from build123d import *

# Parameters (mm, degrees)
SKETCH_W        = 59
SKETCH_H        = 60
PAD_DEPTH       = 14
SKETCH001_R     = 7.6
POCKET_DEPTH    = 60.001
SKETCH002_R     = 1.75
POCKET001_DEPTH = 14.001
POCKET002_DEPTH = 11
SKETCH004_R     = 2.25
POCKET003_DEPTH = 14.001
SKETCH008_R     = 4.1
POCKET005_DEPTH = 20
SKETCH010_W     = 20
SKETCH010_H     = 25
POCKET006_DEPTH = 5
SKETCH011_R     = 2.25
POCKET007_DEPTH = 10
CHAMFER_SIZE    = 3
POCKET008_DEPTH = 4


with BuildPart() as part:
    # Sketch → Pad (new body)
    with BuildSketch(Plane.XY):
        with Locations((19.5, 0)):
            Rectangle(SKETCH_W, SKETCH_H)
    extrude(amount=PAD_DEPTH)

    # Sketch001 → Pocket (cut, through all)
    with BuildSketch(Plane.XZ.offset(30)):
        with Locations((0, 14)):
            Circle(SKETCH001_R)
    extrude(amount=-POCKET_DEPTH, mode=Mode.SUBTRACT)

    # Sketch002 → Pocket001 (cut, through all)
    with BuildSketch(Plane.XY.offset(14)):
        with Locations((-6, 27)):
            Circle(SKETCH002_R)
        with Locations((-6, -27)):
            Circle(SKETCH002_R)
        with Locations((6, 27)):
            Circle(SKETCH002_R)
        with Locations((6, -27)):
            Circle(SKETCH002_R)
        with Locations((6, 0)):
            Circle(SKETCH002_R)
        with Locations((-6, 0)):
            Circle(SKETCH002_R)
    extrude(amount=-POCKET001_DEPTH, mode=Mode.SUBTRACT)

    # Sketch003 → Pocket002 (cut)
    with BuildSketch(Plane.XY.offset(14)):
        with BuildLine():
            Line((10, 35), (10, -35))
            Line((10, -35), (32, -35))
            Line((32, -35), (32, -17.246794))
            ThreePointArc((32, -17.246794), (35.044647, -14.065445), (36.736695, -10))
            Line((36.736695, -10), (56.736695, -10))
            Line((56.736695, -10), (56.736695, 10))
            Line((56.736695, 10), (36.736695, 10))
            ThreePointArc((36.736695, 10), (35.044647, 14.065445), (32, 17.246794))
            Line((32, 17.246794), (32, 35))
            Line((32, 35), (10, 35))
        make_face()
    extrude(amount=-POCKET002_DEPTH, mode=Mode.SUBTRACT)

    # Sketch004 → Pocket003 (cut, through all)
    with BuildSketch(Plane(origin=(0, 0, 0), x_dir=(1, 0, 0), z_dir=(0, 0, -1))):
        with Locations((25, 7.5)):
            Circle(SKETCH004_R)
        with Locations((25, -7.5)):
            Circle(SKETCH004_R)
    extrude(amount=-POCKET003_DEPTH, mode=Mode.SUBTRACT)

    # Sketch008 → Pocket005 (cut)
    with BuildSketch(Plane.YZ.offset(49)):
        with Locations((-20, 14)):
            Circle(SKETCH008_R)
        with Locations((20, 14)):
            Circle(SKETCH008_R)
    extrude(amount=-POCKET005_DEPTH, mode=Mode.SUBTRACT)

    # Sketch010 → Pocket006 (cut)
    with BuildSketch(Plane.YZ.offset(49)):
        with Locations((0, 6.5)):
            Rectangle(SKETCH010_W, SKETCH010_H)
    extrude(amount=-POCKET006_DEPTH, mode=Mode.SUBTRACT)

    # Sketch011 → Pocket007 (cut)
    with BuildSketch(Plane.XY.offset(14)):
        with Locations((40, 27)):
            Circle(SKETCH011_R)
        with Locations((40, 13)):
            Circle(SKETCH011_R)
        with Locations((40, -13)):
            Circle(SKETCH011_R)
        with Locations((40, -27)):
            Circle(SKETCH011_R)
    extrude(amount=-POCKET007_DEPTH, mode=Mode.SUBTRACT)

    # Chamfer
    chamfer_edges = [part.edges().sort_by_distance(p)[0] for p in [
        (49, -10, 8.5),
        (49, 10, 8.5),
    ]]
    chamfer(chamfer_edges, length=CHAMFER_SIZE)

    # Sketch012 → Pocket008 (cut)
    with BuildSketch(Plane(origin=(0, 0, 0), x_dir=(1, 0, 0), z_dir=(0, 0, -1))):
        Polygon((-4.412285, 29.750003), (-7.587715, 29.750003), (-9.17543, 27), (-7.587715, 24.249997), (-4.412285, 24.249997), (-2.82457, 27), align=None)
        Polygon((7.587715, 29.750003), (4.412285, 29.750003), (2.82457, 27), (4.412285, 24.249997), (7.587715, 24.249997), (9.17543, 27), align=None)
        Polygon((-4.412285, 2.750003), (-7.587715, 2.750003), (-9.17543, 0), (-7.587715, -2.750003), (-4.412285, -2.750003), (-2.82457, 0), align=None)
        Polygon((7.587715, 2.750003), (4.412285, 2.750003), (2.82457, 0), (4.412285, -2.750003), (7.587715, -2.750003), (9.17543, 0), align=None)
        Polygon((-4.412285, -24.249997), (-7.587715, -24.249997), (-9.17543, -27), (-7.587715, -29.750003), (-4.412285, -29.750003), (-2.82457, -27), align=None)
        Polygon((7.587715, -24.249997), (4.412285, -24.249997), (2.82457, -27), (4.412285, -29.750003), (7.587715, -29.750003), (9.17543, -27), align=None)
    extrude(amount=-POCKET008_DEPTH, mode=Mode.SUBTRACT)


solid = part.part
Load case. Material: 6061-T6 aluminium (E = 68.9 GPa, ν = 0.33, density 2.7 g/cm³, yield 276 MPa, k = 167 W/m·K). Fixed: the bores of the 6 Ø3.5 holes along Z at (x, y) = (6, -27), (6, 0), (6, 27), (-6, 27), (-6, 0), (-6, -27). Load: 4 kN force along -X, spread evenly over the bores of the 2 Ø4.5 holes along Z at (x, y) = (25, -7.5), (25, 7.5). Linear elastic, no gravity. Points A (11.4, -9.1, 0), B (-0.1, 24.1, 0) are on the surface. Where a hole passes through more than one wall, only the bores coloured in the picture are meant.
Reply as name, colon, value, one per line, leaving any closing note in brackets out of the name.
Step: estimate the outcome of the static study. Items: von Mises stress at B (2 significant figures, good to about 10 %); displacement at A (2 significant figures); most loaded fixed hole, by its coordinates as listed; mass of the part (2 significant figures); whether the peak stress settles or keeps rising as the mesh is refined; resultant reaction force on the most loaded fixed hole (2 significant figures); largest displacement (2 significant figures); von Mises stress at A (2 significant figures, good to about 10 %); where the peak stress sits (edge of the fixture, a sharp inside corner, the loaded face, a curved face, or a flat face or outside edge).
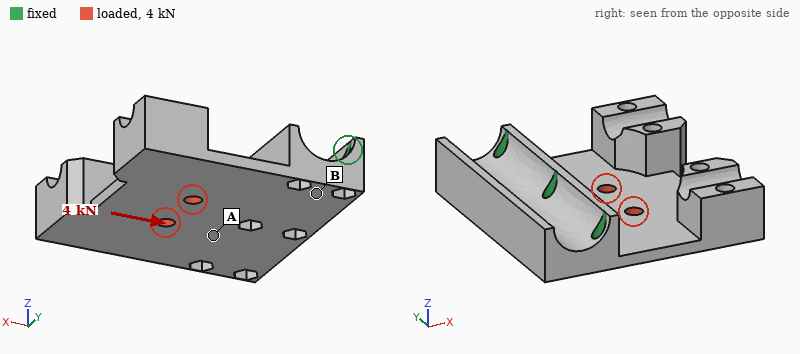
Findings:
von Mises stress at B: 10 MPa
displacement at A: 9.1 µm
most loaded fixed hole, by its coordinates as listed: (6, 0)
mass of the part: 60 g
whether the peak stress settles or keeps rising as the mesh is refined: keeps rising
resultant reaction force on the most loaded fixed hole: 1.3 kN
largest displacement: 42 µm
von Mises stress at A: 33 MPa
where the peak stress sits: edge of the fixture
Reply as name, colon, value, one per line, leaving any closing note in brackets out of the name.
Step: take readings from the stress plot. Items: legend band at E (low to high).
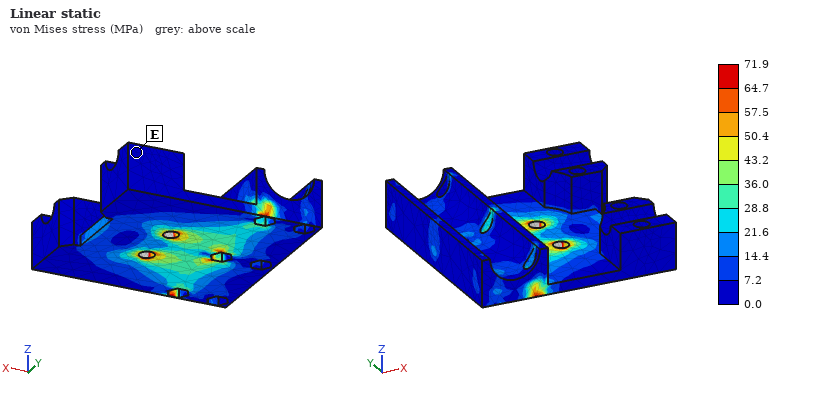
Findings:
legend band at E: 0.0 to 7.2 MPa
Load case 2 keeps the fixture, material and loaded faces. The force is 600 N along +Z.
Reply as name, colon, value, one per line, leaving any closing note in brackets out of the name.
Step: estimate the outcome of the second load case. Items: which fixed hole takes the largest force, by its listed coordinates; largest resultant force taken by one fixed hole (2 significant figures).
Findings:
which fixed hole takes the largest force, by its listed coordinates: (6, 0)
largest resultant force taken by one fixed hole: 830 N
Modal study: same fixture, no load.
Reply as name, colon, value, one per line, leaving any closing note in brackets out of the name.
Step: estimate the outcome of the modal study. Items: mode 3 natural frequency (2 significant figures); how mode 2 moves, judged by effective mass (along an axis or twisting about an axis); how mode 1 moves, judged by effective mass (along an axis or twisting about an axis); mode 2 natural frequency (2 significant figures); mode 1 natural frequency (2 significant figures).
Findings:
mode 3 natural frequency: 3900 Hz
how mode 2 moves, judged by effective mass: twisting about X
how mode 1 moves, judged by effective mass: along Z
mode 2 natural frequency: 1500 Hz
mode 1 natural frequency: 920 Hz
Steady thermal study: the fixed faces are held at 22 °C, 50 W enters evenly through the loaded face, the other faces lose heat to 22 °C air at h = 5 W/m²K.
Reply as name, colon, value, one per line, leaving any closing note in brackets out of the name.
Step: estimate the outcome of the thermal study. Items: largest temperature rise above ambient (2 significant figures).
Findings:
largest temperature rise above ambient: 46 K
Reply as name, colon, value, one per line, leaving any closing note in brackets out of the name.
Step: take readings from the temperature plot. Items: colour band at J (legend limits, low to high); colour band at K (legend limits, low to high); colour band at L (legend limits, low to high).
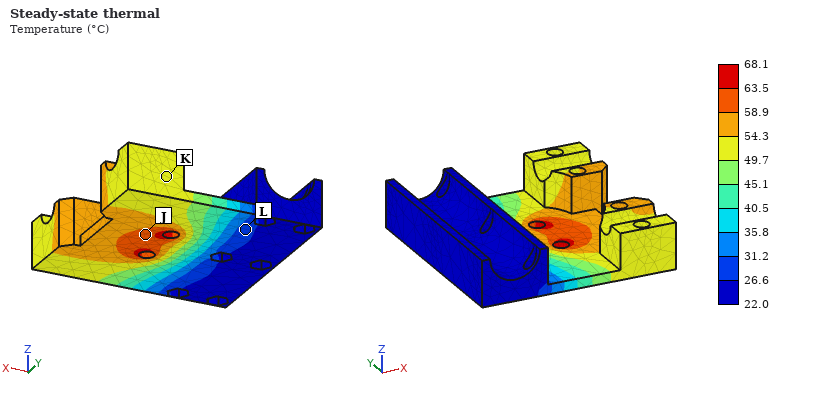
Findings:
colour band at J: 58.9 to 63.5 °C
colour band at K: 49.7 to 54.3 °C
colour band at L: 26.6 to 31.2 °C
